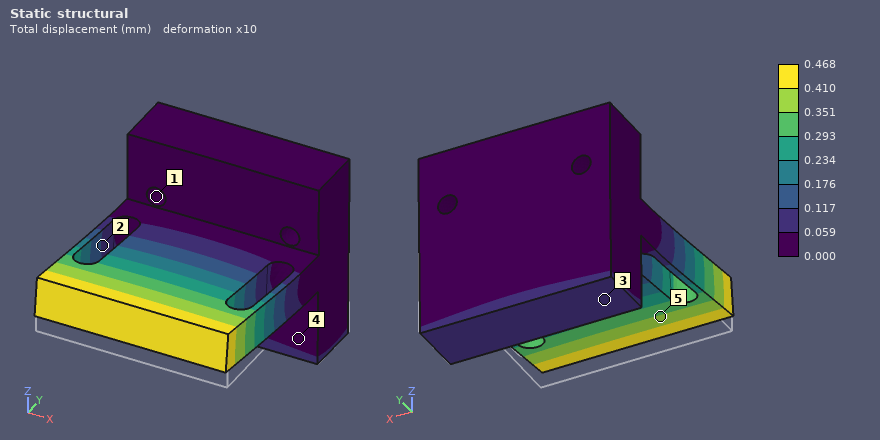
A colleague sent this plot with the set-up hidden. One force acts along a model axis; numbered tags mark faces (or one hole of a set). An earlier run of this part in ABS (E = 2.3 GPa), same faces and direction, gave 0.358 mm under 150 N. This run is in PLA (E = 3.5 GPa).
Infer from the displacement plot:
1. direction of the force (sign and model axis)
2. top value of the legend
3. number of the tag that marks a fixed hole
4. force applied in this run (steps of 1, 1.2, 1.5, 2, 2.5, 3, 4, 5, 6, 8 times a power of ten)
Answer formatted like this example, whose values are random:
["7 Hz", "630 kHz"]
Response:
["+Z", "0.468 mm", "1", "300 N"]
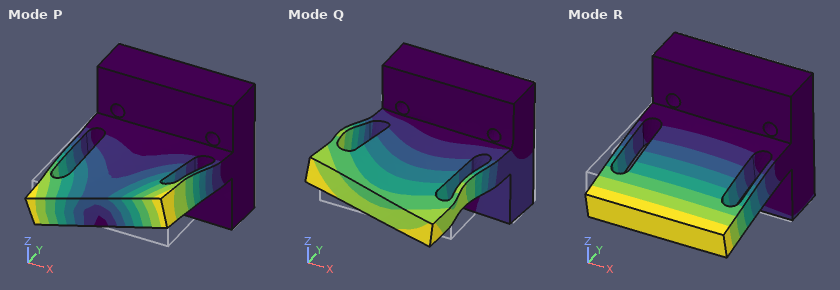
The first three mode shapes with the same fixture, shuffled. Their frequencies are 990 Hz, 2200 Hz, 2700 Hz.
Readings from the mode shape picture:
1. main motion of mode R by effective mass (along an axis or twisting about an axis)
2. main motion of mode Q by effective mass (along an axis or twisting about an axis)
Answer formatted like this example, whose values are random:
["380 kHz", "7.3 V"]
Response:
["along Z", "along X"]
